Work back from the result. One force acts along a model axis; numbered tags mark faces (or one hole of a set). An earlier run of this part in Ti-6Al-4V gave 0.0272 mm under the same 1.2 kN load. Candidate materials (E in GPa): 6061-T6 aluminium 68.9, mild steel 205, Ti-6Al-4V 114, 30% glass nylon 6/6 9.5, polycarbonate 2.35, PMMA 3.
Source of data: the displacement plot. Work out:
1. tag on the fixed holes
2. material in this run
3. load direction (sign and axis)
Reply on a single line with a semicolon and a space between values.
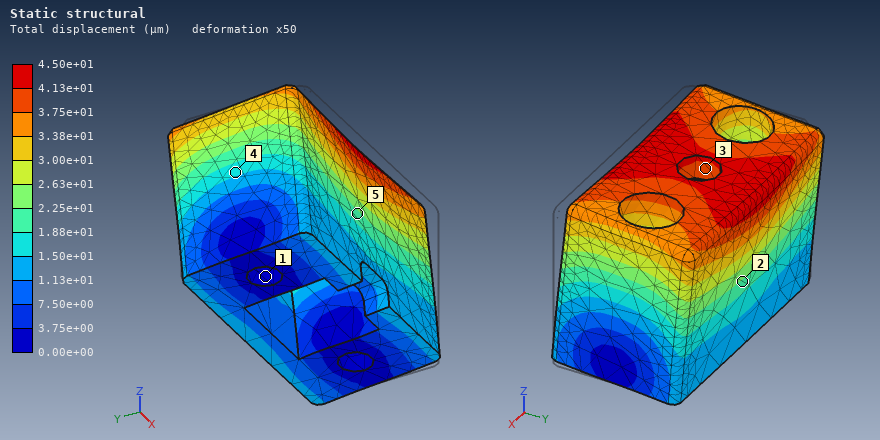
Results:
1; 6061-T6 aluminium; +Y
